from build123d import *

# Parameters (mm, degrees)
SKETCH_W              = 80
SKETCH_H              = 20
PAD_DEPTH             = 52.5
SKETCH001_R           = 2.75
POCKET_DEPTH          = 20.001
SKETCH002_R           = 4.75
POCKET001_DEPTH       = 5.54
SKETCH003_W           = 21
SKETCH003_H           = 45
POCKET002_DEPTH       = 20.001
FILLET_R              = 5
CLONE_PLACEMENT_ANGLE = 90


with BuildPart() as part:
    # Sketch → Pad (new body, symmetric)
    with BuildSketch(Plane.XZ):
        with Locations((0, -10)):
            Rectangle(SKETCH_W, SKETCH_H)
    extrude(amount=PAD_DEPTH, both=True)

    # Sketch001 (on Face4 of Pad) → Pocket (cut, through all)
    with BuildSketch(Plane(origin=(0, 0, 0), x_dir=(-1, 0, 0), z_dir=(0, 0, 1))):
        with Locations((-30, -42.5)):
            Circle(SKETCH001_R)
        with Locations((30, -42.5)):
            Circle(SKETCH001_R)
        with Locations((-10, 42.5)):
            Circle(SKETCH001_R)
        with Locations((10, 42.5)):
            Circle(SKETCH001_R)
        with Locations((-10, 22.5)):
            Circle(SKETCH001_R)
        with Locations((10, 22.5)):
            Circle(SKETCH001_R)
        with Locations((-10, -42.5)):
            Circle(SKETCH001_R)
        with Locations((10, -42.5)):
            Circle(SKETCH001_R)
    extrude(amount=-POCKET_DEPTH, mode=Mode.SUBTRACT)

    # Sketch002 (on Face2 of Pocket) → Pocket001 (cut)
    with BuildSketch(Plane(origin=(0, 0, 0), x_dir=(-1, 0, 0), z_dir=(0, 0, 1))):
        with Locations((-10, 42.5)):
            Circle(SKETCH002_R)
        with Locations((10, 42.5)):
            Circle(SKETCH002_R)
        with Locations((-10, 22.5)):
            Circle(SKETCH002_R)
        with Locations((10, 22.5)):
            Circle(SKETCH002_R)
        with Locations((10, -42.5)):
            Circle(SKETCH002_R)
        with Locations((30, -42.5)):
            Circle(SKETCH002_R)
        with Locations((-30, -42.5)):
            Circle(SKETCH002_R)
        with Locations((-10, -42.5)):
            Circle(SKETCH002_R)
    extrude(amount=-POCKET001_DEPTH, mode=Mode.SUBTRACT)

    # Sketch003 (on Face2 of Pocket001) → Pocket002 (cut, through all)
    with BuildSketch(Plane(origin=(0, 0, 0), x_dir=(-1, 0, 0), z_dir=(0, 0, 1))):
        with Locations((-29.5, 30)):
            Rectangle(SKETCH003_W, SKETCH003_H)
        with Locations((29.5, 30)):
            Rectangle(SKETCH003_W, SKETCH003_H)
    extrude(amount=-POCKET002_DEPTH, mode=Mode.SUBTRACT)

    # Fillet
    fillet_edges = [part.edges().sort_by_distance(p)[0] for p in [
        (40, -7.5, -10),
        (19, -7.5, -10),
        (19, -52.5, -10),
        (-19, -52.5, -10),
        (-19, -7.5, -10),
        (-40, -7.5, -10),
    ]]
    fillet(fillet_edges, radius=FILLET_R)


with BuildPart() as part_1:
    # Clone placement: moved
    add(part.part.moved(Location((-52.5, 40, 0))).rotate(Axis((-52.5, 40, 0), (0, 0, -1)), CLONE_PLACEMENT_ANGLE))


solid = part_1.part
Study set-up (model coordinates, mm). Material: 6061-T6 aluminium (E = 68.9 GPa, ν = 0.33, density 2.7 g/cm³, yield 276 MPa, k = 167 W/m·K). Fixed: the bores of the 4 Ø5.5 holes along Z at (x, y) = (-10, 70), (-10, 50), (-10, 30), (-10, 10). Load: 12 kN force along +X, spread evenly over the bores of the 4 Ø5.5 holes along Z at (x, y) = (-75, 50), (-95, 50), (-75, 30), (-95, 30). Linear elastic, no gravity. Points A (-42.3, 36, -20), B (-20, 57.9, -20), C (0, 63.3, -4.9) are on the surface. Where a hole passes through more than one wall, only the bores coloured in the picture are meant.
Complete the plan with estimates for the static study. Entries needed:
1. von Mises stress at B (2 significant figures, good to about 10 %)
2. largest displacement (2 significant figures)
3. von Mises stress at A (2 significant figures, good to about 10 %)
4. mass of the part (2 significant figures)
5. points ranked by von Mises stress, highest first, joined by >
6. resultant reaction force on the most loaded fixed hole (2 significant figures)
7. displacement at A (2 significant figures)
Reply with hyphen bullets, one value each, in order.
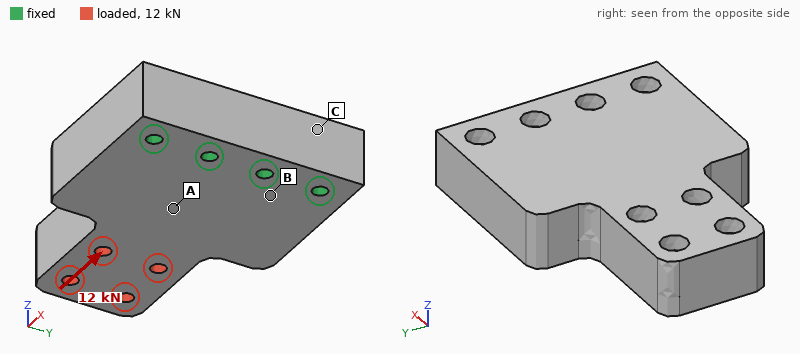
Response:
- 11 MPa
- 53 µm
- 20 MPa
- 340 g
- A > B > C
- 3.1 kN
- 8.9 µm
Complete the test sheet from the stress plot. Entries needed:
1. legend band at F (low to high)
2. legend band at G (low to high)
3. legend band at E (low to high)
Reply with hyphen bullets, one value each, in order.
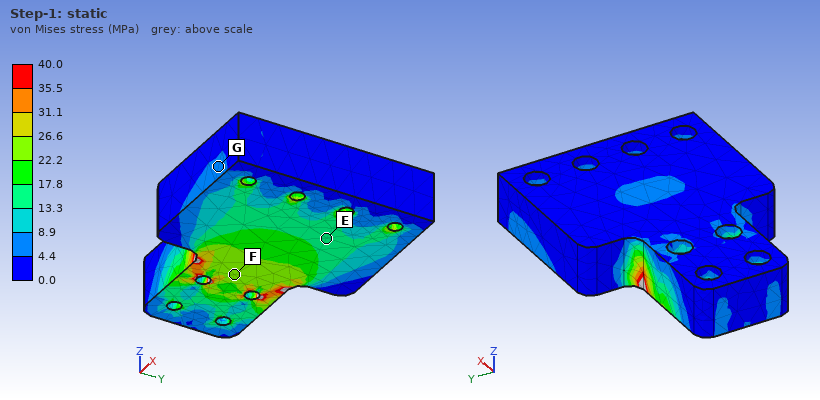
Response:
- 22.2 to 26.6 MPa
- 4.4 to 8.9 MPa
- 13.3 to 17.8 MPa
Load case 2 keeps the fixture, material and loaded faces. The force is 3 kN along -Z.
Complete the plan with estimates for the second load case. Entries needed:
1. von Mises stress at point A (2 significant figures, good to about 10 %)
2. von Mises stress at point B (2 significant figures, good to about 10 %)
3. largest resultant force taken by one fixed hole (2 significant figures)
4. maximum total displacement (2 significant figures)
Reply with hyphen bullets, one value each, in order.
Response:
- 30 MPa
- 34 MPa
- 1.3 kN
- 0.26 mm
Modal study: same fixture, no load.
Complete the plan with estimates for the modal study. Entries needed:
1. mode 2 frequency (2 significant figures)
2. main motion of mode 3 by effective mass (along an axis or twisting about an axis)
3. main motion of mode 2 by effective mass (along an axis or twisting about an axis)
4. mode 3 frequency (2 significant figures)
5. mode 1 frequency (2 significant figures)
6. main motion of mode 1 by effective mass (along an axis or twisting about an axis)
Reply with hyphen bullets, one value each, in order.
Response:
- 5900 Hz
- twisting about X
- along Y
- 7100 Hz
- 2100 Hz
- along Z
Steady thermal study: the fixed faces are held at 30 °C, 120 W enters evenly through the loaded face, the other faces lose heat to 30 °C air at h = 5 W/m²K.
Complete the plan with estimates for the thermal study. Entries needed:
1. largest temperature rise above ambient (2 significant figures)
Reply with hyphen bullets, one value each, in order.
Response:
- 56 K
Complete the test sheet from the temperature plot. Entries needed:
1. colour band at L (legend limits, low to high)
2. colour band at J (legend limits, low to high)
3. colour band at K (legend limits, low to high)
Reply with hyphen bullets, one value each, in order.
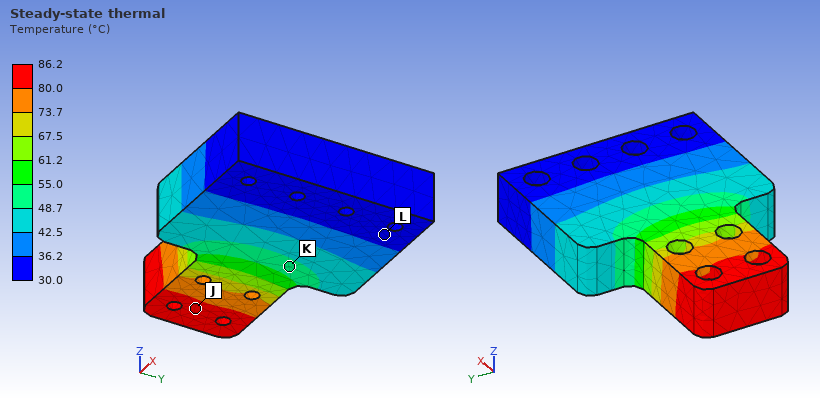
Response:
- 30.0 to 36.2 °C
- 80.0 to 86.2 °C
- 48.7 to 55.0 °C
